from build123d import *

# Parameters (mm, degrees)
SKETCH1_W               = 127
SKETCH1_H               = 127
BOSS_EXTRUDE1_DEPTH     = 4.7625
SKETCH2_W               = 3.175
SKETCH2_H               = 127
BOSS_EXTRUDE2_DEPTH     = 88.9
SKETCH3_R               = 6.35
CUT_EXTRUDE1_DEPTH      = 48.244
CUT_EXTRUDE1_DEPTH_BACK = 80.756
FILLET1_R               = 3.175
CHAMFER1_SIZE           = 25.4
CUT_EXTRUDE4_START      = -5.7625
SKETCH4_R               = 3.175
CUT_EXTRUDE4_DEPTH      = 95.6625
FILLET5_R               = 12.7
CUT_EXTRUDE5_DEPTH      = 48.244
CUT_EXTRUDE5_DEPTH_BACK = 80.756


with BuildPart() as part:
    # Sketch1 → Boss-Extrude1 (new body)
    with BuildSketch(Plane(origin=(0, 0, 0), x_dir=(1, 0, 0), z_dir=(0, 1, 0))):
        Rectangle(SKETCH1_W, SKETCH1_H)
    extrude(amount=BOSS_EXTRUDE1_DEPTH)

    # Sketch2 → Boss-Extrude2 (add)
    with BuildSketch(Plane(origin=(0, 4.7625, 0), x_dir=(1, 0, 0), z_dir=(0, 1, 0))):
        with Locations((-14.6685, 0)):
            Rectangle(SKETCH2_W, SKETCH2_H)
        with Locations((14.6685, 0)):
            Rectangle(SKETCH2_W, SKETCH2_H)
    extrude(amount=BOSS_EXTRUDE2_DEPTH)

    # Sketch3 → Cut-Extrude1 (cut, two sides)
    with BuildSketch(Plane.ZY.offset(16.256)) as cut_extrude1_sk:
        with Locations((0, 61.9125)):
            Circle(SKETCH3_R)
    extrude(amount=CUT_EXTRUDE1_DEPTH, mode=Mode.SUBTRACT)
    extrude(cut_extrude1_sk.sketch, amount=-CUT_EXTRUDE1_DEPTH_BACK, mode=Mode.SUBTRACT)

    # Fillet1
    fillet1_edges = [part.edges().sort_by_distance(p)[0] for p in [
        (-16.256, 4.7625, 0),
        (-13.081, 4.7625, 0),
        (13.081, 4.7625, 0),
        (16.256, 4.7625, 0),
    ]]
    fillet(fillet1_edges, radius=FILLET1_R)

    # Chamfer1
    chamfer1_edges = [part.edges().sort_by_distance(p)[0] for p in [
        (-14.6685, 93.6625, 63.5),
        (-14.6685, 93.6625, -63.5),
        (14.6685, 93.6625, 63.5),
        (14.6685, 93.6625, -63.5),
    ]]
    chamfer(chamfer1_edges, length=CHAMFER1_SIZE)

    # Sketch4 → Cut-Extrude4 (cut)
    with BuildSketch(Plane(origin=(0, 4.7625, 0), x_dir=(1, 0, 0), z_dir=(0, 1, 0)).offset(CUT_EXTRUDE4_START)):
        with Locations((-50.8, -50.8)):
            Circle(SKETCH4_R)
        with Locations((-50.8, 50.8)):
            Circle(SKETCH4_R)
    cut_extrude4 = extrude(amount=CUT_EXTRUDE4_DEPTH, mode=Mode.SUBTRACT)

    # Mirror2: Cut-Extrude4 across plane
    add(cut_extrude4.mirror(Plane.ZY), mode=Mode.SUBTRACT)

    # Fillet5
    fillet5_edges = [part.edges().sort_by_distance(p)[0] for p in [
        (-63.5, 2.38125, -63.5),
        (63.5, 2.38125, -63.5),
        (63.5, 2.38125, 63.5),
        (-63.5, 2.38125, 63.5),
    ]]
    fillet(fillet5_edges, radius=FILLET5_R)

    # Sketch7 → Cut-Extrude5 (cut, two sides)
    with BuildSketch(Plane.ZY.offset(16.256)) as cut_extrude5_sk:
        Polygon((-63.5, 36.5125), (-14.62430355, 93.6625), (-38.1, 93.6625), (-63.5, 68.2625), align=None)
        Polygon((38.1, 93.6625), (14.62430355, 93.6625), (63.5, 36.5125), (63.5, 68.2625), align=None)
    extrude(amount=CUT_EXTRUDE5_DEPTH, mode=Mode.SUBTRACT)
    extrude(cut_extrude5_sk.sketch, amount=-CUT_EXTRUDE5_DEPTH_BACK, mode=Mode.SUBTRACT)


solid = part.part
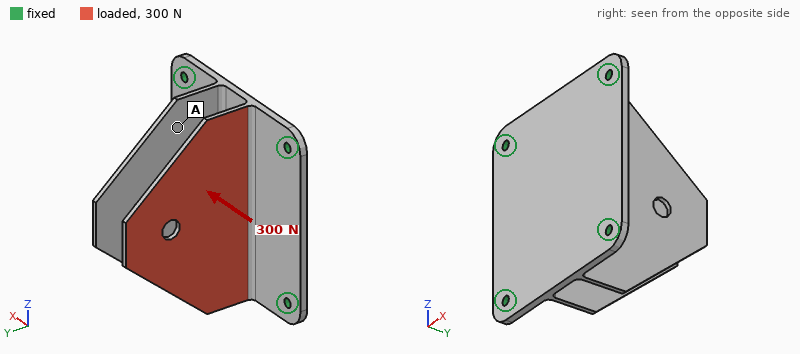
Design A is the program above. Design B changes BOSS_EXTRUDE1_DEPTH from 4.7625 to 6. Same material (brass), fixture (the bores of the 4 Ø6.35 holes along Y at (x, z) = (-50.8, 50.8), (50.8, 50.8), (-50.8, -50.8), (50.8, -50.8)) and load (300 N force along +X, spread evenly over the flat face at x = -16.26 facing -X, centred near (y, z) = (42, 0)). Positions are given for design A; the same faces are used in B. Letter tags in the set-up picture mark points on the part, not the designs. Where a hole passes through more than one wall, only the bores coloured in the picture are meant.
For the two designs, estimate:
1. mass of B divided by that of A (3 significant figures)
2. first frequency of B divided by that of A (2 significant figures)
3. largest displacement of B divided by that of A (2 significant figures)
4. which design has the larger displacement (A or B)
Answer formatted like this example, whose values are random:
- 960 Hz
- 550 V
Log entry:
- 1.14
- 1.1
- 0.92
- A
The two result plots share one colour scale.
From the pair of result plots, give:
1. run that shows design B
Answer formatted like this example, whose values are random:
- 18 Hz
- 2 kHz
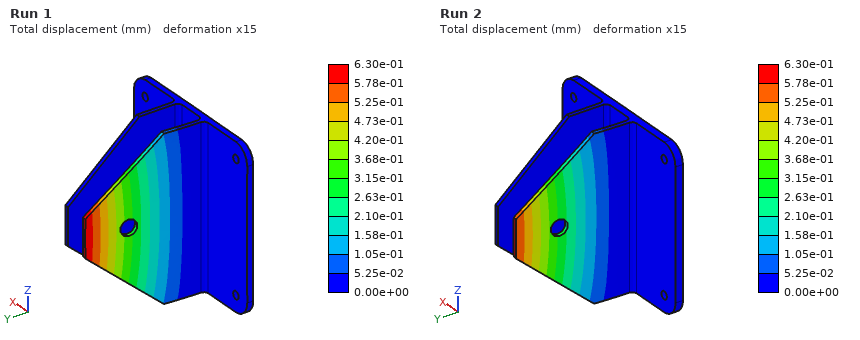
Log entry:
- Run 2
